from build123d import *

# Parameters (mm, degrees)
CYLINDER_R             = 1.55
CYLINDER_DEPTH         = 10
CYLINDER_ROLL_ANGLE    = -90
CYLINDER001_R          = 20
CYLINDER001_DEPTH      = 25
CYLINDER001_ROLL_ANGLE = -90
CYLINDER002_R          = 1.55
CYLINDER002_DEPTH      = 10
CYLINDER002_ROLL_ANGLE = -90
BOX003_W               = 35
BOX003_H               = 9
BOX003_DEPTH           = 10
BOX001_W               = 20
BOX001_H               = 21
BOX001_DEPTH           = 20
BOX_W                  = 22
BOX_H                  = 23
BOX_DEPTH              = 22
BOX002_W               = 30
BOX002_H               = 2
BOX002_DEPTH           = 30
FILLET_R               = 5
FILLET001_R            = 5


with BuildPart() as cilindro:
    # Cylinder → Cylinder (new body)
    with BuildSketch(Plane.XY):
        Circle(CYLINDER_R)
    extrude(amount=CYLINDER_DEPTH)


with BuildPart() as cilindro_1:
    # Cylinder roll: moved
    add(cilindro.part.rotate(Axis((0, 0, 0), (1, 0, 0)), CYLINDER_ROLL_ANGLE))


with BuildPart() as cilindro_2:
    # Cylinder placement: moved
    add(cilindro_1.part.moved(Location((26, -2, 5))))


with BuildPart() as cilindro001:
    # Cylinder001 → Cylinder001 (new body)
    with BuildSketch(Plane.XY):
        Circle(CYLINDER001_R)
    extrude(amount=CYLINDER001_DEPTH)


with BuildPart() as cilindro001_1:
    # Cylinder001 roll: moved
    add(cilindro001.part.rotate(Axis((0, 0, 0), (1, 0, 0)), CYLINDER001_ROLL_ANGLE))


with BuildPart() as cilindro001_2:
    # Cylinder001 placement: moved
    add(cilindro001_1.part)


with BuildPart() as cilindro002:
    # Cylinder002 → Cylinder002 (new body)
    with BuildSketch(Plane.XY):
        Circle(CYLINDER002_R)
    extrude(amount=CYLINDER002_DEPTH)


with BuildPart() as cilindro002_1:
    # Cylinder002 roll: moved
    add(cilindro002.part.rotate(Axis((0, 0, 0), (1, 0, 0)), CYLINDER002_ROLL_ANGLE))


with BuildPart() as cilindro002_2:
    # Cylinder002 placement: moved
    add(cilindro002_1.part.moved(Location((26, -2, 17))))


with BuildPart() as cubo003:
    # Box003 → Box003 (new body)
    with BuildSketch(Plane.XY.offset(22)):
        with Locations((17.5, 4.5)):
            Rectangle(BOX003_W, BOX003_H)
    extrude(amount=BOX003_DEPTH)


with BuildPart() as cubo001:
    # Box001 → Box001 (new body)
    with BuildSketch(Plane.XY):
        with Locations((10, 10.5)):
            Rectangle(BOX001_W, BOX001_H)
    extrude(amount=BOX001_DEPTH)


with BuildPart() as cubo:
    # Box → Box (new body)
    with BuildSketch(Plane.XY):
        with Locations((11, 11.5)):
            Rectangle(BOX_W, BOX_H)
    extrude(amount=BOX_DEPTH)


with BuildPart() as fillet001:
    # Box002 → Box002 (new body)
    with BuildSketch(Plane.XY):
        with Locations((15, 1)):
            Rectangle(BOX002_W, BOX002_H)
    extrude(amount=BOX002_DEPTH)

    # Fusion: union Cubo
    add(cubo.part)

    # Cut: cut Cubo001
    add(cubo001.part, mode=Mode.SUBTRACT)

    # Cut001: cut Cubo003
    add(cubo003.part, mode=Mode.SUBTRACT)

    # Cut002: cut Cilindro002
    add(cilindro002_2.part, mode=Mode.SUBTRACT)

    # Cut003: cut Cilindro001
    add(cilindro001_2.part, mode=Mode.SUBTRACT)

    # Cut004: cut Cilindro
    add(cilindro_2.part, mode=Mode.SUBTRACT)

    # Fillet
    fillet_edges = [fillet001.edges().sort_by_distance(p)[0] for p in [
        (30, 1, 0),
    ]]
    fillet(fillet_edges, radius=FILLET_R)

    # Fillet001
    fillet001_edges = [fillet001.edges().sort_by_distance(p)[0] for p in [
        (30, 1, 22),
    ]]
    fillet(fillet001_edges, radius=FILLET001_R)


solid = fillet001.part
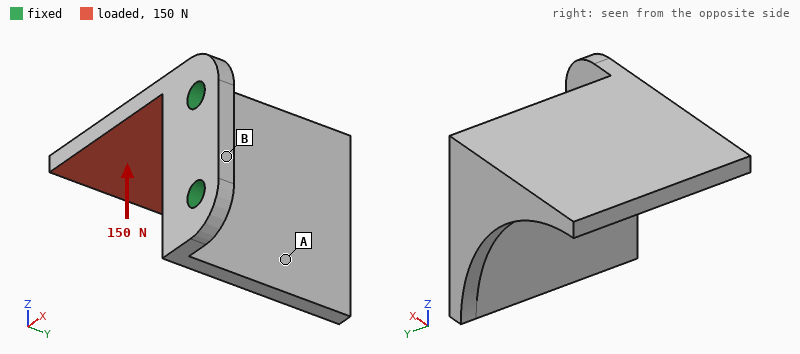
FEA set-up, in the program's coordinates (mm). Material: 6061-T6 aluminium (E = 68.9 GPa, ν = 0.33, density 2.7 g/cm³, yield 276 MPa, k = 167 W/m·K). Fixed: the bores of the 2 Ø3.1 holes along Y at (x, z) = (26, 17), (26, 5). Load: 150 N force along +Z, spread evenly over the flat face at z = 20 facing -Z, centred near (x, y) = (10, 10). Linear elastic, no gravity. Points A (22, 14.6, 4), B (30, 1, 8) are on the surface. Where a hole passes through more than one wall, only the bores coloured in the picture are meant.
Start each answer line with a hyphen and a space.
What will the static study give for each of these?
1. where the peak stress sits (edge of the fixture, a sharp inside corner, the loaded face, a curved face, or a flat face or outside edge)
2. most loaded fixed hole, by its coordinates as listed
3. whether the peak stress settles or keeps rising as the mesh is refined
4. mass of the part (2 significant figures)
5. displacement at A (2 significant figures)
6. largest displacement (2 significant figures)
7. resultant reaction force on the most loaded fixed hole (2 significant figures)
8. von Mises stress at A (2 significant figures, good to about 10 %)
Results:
- a sharp inside corner
- (26, 5)
- keeps rising
- 6.5 g
- 0.039 mm
- 0.25 mm
- 210 N
- 33 MPa
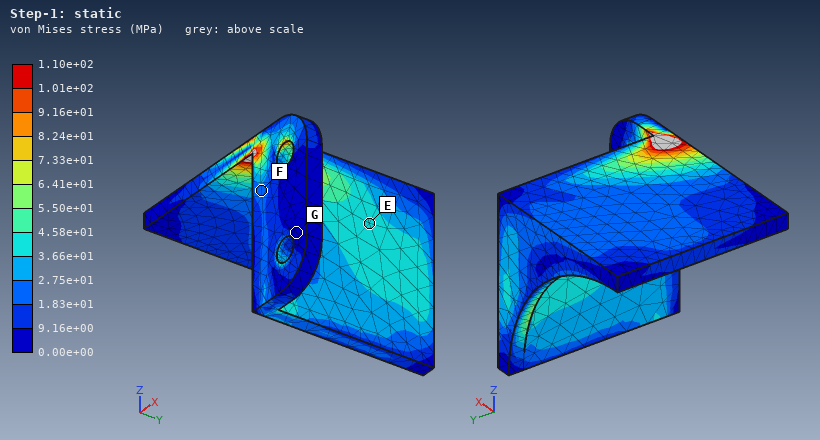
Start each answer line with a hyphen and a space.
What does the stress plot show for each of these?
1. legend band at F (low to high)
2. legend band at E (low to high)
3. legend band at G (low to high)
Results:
- 1.83e+01 to 2.75e+01 MPa
- 3.66e+01 to 4.58e+01 MPa
- 0.00e+00 to 9.16e+00 MPa
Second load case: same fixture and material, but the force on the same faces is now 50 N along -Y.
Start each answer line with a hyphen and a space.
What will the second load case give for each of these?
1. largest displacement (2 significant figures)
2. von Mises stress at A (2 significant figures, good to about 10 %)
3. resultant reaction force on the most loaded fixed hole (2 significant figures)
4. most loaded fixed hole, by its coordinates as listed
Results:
- 0.18 mm
- 10 MPa
- 60 N
- (26, 17)
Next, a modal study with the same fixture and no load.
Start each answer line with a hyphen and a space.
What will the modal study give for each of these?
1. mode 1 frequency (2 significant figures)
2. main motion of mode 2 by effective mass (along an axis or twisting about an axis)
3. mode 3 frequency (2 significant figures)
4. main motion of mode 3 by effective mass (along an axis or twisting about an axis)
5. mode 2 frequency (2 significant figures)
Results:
- 1500 Hz
- along Z
- 6700 Hz
- along Z
- 3000 Hz
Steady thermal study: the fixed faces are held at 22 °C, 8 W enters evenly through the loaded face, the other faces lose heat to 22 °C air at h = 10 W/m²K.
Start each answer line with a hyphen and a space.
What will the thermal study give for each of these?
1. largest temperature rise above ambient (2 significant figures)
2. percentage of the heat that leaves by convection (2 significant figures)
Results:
- 24 K
- 3.5 %
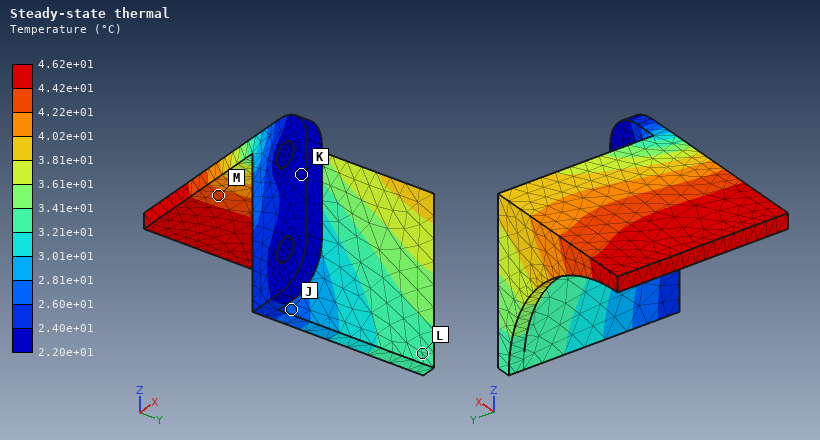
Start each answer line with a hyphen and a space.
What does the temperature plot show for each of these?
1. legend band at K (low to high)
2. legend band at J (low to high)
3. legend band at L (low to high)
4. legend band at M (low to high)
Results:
- 2.20e+01 to 2.40e+01 °C
- 2.60e+01 to 2.81e+01 °C
- 3.21e+01 to 3.41e+01 °C
- 4.22e+01 to 4.42e+01 °C
